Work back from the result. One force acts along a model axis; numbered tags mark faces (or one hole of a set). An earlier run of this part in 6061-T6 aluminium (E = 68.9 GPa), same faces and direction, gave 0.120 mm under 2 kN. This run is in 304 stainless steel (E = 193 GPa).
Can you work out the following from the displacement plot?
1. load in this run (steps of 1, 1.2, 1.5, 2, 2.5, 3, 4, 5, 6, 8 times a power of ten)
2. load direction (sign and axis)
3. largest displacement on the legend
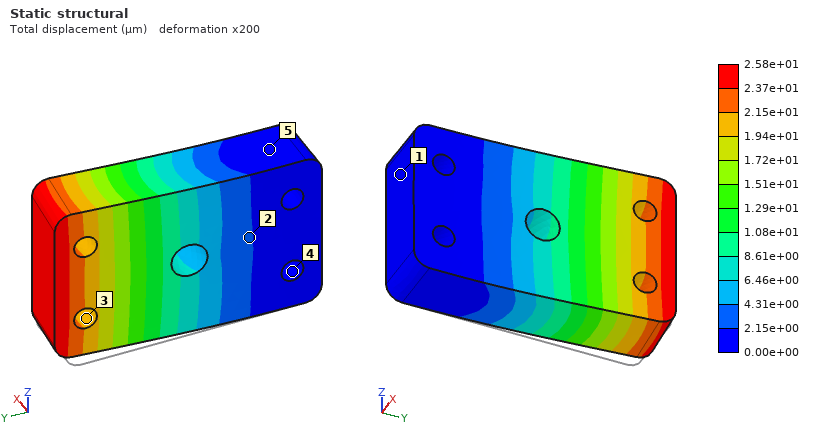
1.2 kN
+X
2.58e+01 µm
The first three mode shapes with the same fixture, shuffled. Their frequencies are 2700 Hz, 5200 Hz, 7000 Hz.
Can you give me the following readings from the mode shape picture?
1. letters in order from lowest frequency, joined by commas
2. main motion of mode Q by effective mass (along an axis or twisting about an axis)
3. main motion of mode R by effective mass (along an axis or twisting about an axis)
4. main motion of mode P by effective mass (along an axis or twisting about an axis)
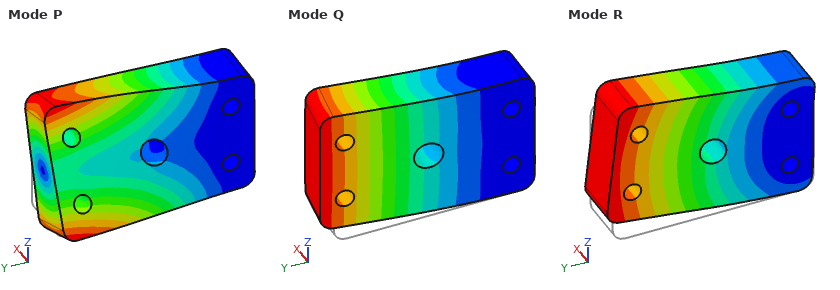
Q, R, P
along X
along Z
twisting about Y
